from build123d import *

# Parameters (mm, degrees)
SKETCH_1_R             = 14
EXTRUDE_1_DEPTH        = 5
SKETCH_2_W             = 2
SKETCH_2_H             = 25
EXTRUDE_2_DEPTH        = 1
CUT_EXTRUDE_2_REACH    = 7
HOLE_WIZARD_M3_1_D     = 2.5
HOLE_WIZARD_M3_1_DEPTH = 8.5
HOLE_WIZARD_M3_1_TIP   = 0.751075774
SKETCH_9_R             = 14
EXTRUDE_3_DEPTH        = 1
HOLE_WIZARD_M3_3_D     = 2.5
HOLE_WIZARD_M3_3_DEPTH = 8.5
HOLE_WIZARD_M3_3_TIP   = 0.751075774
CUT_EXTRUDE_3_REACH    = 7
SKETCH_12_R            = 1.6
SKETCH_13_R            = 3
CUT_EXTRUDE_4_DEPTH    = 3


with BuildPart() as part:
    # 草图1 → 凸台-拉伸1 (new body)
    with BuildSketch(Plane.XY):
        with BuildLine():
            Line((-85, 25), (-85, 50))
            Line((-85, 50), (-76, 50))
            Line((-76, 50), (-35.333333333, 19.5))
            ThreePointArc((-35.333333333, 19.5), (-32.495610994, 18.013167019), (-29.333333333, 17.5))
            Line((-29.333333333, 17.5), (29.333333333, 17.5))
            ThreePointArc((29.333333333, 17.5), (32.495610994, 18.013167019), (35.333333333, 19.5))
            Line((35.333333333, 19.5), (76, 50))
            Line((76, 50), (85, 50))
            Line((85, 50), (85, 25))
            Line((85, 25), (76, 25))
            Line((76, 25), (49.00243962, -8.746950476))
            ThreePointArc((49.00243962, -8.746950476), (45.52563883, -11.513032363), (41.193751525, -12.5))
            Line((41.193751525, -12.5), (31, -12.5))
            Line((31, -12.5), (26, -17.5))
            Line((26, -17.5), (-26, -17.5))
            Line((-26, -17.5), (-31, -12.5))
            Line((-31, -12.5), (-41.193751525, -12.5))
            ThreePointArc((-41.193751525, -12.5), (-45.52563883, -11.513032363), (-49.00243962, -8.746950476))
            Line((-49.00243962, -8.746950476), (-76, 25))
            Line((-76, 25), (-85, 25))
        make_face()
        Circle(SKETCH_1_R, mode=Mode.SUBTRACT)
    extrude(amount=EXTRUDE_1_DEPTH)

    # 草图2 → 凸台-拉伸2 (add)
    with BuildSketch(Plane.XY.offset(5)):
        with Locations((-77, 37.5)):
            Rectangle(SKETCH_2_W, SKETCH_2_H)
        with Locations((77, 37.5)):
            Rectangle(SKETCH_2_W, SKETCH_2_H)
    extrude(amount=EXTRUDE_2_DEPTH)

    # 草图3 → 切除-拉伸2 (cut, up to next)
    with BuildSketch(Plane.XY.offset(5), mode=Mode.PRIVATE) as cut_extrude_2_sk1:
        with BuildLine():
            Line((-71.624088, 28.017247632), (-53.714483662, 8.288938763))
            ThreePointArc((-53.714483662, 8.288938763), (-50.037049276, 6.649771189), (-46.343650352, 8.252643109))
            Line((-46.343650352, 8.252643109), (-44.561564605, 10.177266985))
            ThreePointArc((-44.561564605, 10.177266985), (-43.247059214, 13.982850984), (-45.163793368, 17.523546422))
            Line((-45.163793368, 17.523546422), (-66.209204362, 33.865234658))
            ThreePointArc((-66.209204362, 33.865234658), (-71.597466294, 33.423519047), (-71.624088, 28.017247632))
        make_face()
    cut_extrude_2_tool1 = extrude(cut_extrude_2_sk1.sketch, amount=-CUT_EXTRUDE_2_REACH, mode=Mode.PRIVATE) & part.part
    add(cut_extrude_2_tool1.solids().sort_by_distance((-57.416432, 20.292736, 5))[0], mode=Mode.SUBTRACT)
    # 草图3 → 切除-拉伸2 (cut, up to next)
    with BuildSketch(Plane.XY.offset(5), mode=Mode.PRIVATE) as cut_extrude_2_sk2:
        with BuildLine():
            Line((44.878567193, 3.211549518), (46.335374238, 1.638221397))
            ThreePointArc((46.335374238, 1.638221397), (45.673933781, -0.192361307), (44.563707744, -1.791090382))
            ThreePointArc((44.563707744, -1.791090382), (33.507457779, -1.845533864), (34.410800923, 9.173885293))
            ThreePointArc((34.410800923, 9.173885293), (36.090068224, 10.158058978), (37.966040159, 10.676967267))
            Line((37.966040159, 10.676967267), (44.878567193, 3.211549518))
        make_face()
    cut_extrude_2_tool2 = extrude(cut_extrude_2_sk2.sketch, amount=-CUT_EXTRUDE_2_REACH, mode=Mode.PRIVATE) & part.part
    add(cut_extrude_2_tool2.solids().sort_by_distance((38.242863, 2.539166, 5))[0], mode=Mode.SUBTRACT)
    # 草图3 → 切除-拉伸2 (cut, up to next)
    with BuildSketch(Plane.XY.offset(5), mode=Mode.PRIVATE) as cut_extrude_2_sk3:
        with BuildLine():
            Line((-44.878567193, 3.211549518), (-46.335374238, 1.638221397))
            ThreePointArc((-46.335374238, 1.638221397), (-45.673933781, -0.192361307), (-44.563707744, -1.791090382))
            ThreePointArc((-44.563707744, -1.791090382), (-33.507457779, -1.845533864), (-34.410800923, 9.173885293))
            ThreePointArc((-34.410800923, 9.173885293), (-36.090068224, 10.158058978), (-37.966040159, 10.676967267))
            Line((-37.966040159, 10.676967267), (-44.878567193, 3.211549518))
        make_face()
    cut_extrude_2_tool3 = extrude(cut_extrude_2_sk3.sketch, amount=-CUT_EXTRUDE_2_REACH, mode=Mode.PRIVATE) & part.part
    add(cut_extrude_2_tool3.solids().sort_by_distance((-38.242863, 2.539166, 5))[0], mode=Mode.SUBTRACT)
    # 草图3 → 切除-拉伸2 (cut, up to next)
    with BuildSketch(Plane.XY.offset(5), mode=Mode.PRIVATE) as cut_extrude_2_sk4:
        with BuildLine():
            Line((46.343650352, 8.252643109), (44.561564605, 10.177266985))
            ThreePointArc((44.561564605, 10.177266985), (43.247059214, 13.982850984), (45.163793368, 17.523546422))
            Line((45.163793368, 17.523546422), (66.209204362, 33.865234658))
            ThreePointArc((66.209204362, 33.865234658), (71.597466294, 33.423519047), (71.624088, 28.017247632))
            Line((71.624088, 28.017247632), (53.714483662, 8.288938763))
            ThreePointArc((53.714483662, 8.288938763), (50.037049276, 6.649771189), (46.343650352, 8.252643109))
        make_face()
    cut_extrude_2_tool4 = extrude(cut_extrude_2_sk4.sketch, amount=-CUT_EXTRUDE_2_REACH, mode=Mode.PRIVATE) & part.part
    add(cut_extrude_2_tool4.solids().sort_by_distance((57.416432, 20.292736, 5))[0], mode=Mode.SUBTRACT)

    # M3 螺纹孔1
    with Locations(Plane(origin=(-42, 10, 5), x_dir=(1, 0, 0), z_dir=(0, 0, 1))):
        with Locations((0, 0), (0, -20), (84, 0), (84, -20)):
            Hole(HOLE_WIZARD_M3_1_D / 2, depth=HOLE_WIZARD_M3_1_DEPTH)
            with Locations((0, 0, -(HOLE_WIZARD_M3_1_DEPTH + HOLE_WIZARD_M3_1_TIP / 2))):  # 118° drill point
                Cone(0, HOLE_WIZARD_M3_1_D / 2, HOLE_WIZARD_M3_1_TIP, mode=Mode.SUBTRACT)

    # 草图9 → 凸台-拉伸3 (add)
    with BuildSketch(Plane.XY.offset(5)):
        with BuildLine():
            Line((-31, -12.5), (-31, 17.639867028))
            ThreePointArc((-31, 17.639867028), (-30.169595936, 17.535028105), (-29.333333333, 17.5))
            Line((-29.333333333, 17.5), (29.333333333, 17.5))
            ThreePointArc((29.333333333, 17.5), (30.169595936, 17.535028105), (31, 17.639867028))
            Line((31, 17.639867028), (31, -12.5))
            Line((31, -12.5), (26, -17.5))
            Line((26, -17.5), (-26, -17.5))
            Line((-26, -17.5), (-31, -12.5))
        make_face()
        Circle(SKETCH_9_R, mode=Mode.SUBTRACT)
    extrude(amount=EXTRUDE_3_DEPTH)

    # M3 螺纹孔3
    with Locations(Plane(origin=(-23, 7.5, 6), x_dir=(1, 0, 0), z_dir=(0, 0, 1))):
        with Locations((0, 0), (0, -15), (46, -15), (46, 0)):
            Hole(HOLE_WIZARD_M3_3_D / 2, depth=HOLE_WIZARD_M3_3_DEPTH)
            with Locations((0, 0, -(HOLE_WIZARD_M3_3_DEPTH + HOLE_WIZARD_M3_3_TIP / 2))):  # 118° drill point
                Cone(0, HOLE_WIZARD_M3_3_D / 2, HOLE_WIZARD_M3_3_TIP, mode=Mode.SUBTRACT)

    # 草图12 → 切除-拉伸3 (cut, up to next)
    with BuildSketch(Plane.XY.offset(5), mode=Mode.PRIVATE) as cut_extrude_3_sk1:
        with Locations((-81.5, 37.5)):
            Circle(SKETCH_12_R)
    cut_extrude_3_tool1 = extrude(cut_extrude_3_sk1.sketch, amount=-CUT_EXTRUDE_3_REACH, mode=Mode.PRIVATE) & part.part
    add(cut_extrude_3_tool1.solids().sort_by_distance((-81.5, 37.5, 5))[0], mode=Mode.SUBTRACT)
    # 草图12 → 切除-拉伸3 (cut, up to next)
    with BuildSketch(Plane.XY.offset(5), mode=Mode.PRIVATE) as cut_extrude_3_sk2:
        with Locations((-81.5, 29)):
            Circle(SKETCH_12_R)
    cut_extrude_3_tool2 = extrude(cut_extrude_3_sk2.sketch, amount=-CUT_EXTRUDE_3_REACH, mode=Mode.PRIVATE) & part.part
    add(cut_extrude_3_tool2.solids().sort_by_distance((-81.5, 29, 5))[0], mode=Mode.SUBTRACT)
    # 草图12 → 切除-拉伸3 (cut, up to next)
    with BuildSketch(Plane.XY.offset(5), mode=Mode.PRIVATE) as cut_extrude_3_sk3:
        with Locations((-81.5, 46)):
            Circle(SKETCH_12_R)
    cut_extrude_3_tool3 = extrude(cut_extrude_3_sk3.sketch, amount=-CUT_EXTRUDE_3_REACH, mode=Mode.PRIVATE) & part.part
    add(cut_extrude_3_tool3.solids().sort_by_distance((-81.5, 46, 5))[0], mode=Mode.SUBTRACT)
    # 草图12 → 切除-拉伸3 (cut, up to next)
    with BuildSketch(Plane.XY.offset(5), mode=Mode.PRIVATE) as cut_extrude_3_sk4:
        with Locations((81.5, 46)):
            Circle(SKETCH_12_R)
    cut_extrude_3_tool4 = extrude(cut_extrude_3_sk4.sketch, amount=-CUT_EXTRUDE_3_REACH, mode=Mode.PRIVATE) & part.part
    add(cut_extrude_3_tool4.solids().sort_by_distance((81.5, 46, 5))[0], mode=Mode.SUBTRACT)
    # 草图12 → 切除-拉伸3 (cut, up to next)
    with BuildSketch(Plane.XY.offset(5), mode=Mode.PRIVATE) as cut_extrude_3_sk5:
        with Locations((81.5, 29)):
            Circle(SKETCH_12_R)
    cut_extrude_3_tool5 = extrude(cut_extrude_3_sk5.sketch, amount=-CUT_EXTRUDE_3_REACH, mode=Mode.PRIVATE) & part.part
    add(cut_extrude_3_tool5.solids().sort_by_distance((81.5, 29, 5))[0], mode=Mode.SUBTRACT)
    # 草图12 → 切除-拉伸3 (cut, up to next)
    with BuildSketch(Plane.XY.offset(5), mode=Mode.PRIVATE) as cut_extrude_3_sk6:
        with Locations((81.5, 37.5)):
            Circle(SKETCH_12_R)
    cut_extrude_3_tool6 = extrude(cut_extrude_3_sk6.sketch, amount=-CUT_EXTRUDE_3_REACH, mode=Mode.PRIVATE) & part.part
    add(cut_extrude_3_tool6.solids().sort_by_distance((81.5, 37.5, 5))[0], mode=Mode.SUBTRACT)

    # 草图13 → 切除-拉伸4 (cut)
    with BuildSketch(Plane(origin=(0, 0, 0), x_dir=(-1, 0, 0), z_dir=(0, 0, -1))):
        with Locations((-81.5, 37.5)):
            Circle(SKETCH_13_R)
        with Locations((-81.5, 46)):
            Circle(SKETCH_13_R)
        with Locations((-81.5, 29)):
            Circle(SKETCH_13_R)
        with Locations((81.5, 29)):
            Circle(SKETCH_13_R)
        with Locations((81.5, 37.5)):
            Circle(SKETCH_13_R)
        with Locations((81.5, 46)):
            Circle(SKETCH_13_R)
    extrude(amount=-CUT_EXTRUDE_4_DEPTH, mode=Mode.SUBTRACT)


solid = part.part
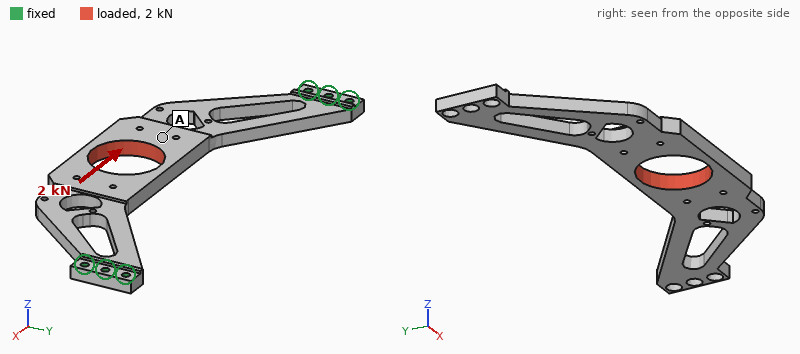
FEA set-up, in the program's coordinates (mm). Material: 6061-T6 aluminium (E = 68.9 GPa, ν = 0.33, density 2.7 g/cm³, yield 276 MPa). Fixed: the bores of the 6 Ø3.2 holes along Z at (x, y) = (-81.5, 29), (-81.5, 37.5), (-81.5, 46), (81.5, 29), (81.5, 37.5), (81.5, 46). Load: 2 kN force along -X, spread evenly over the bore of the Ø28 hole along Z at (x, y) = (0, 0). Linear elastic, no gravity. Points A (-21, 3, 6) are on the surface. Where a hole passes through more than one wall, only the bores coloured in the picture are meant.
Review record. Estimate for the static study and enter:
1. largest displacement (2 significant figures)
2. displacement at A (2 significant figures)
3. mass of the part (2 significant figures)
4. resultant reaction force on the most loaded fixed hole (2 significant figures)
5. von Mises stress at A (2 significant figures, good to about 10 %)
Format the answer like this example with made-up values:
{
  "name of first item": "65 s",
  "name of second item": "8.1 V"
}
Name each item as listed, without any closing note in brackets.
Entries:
{
  "largest displacement": "78 µm",
  "displacement at A": "73 µm",
  "mass of the part": "56 g",
  "resultant reaction force on the most loaded fixed hole": "480 N",
  "von Mises stress at A": "11 MPa"
}
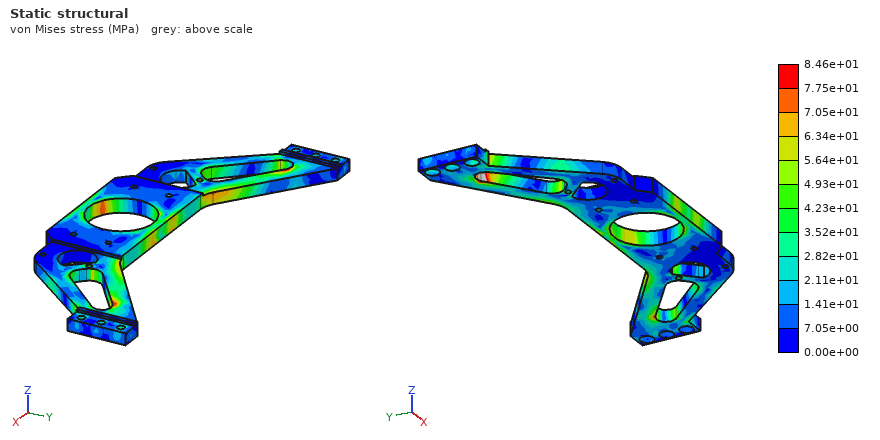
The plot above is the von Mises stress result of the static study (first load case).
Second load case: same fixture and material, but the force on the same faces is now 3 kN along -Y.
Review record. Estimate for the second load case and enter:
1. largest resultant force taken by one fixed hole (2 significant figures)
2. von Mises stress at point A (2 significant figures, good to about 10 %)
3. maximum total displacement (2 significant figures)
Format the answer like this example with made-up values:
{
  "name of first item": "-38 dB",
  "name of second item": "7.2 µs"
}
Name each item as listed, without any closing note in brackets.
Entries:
{
  "largest resultant force taken by one fixed hole": "1.3 kN",
  "von Mises stress at point A": "20 MPa",
  "maximum total displacement": "0.17 mm"
}
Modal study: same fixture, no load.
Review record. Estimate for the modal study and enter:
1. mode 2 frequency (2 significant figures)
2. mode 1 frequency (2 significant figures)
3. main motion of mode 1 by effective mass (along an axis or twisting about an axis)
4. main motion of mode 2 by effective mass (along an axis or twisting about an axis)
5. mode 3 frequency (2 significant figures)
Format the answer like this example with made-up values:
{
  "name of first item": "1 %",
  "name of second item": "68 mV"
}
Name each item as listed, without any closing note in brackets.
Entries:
{
  "mode 2 frequency": "1600 Hz",
  "mode 1 frequency": "510 Hz",
  "main motion of mode 1 by effective mass": "along Z",
  "main motion of mode 2 by effective mass": "twisting about Y",
  "mode 3 frequency": "1900 Hz"
}
